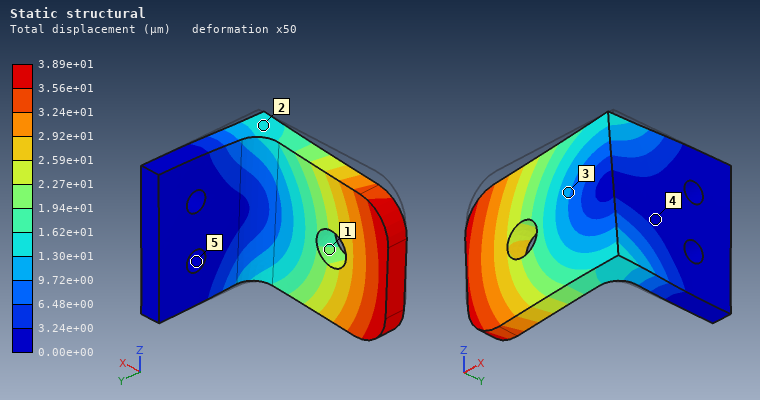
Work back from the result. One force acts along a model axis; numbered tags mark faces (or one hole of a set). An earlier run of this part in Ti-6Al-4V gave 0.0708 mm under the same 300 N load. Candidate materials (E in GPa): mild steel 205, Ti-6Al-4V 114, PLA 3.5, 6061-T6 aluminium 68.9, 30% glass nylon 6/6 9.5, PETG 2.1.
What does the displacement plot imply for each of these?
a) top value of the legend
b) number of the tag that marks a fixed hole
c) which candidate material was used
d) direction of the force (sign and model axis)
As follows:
3.89e+01 µm
5
mild steel
-Z
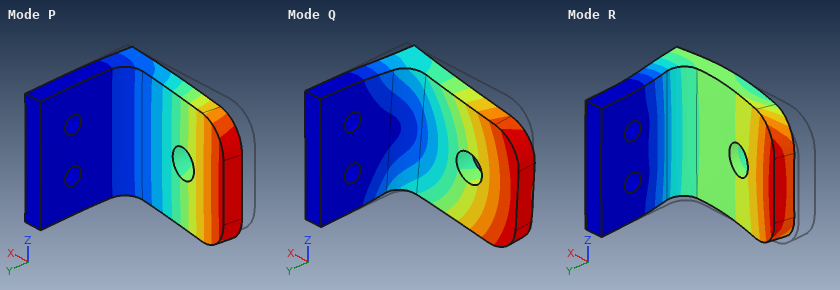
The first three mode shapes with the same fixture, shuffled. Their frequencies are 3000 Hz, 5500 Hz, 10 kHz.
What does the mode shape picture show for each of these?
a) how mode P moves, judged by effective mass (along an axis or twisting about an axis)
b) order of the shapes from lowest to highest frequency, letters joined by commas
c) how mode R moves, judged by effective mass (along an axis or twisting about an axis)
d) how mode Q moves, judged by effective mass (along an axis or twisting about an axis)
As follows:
along Y
P, Q, R
along X
along Z
